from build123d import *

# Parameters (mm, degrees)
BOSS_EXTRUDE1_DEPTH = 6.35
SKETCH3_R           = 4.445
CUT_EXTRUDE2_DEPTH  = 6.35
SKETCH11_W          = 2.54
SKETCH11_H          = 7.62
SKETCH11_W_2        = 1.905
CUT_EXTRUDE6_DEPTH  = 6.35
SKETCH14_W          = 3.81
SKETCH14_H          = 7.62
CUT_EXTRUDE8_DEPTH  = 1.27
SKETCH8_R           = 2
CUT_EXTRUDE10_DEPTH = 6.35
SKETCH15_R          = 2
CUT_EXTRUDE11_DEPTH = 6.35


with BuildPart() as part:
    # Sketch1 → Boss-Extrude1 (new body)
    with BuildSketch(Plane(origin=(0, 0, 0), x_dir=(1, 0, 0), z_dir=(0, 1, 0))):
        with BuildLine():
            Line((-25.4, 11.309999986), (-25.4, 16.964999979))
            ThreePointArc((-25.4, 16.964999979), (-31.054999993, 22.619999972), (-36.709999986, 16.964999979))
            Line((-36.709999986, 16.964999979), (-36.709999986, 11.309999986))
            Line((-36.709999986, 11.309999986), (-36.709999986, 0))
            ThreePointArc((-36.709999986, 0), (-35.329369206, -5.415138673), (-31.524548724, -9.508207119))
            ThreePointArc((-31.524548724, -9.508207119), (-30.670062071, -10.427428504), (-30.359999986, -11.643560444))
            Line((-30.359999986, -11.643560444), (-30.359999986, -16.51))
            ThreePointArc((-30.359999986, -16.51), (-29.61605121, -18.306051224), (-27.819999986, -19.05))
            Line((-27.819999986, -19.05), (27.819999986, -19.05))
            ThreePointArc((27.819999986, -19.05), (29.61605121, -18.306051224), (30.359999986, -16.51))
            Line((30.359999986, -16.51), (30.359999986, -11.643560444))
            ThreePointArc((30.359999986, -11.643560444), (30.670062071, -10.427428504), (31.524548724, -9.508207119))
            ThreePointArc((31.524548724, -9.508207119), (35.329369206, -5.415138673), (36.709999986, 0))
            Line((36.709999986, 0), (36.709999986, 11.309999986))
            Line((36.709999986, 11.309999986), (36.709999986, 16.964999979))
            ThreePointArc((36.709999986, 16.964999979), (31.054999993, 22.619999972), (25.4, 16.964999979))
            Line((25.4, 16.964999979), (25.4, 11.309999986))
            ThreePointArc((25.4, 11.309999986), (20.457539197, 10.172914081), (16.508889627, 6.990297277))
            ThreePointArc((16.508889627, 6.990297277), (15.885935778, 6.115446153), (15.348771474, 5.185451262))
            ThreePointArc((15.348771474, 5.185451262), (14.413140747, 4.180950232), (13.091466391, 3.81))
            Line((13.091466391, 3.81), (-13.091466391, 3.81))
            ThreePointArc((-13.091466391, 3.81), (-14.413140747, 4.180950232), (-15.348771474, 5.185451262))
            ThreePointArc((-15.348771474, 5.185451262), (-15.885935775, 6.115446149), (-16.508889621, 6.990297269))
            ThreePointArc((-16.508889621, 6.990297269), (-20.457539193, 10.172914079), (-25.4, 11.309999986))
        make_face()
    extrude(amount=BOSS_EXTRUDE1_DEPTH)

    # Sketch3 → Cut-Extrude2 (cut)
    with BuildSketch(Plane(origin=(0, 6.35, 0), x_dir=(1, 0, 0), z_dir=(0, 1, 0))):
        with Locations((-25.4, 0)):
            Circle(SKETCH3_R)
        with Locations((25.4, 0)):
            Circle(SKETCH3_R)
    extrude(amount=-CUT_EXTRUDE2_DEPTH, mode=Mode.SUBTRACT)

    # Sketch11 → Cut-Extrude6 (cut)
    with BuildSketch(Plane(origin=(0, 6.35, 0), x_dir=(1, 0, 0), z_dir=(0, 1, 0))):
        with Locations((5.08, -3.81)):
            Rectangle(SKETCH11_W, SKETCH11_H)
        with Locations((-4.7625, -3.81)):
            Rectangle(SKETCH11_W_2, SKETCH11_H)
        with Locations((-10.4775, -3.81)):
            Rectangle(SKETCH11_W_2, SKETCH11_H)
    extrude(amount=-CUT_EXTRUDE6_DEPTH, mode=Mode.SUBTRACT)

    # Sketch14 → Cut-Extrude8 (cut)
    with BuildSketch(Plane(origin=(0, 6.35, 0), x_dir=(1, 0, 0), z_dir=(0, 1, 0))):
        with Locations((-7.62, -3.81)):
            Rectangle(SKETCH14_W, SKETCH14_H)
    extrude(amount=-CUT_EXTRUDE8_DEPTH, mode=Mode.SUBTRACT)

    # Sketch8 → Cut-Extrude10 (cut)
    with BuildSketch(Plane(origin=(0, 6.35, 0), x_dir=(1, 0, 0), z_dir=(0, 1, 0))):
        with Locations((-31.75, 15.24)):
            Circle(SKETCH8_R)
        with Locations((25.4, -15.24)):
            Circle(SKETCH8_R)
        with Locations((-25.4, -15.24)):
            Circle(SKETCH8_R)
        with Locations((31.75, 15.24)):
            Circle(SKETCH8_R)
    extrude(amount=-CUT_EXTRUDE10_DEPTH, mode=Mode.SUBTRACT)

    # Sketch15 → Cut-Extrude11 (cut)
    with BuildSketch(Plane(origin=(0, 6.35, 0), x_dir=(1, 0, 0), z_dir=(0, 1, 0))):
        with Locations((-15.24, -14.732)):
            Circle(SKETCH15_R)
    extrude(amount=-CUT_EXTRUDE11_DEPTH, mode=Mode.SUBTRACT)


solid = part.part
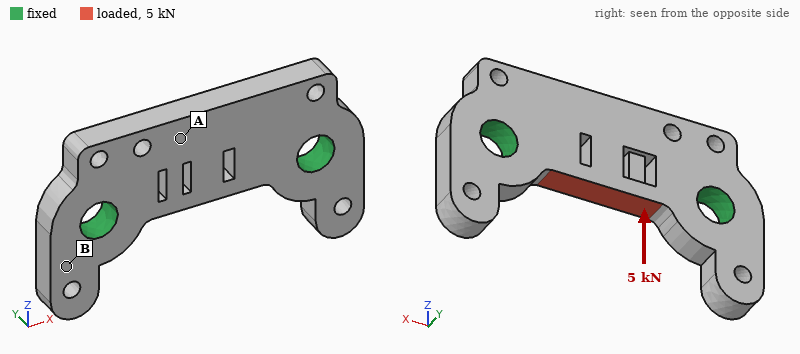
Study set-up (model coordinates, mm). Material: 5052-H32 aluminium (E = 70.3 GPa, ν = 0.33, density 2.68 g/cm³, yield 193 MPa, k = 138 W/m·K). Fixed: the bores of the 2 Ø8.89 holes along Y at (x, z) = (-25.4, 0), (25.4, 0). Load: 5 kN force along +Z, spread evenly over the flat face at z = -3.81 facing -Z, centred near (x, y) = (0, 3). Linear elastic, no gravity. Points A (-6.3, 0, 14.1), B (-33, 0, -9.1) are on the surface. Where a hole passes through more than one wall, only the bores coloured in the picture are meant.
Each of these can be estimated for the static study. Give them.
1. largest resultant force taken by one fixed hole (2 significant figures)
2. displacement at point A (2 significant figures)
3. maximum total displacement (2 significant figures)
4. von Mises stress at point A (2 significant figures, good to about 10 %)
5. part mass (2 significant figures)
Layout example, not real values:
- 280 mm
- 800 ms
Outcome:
- 2.8 kN
- 18 µm
- 28 µm
- 37 MPa
- 31 g
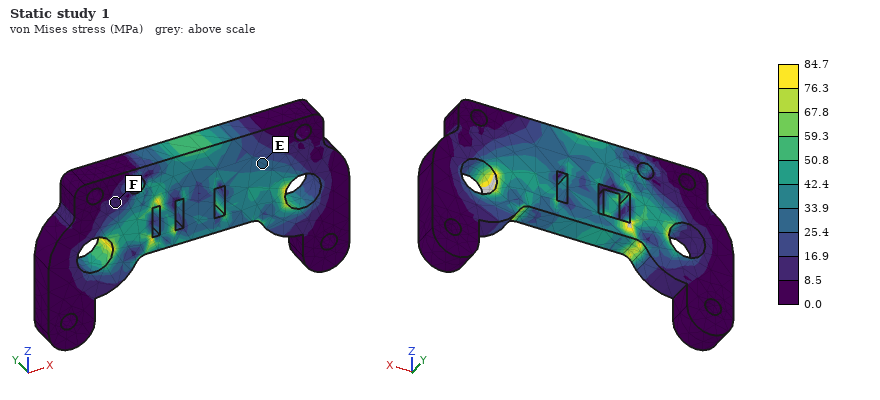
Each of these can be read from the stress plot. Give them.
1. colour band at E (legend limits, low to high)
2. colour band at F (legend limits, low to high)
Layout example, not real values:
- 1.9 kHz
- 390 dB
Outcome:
- 25.4 to 33.9 MPa
- 8.5 to 16.9 MPa
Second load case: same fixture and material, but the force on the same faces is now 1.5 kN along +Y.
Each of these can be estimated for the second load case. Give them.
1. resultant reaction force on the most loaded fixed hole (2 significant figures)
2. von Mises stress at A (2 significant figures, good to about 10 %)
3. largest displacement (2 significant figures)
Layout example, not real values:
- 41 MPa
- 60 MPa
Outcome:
- 760 N
- 18 MPa
- 52 µm
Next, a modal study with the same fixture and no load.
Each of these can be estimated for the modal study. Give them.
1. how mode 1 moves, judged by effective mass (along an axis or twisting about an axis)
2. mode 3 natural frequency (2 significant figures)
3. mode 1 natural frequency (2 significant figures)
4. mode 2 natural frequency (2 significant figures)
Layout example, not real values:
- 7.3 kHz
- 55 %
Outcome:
- along Y
- 15 kHz
- 10 kHz
- 15 kHz
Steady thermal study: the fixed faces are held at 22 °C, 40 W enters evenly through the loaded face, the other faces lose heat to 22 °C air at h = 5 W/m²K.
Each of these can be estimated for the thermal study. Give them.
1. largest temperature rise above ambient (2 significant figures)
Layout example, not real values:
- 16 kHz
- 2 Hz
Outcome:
- 33 K
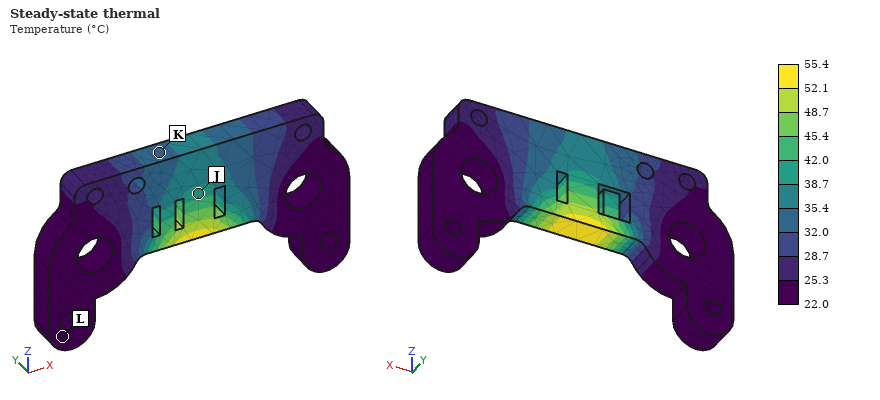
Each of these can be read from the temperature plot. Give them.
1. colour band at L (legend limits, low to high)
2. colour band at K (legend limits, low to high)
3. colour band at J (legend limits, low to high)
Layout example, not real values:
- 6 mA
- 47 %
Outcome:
- 22.0 to 25.3 °C
- 32.0 to 35.4 °C
- 38.7 to 42.0 °C
